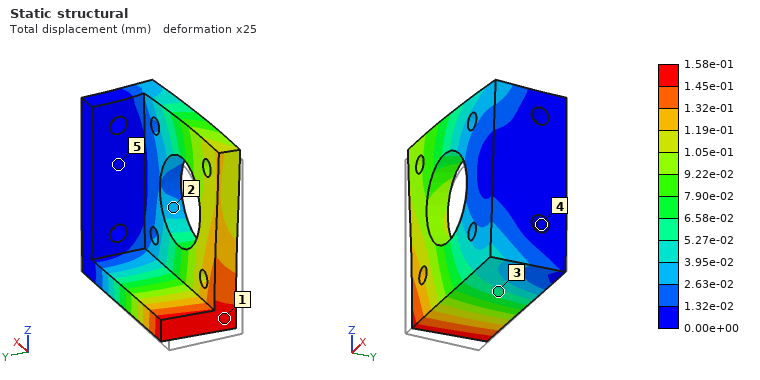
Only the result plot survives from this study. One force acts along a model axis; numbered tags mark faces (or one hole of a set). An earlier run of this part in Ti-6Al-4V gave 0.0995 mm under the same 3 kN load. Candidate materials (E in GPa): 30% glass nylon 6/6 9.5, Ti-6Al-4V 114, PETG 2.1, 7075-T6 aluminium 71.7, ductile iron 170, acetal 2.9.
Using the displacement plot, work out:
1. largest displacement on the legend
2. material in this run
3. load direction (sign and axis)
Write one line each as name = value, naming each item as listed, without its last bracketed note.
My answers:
largest displacement on the legend = 1.58e-01 mm
material in this run = 7075-T6 aluminium
load direction = +Z
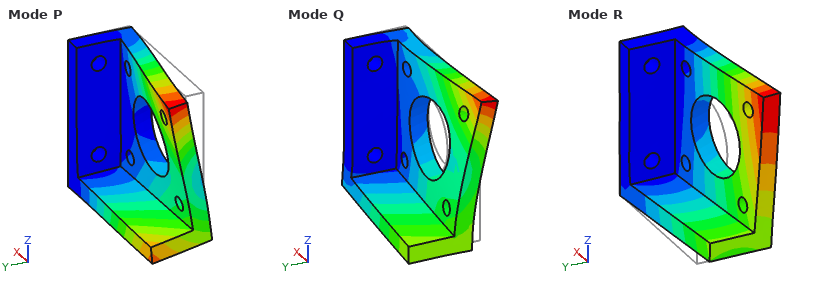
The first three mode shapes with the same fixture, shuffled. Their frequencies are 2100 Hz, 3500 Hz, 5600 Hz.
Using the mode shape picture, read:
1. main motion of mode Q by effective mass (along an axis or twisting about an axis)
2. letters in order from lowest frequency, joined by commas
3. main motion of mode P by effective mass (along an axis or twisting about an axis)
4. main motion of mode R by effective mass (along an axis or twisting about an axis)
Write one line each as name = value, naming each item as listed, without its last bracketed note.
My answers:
main motion of mode Q by effective mass = along Z
letters in order from lowest frequency, joined by commas = R, P, Q
main motion of mode P by effective mass = along Z
main motion of mode R by effective mass = along Y
